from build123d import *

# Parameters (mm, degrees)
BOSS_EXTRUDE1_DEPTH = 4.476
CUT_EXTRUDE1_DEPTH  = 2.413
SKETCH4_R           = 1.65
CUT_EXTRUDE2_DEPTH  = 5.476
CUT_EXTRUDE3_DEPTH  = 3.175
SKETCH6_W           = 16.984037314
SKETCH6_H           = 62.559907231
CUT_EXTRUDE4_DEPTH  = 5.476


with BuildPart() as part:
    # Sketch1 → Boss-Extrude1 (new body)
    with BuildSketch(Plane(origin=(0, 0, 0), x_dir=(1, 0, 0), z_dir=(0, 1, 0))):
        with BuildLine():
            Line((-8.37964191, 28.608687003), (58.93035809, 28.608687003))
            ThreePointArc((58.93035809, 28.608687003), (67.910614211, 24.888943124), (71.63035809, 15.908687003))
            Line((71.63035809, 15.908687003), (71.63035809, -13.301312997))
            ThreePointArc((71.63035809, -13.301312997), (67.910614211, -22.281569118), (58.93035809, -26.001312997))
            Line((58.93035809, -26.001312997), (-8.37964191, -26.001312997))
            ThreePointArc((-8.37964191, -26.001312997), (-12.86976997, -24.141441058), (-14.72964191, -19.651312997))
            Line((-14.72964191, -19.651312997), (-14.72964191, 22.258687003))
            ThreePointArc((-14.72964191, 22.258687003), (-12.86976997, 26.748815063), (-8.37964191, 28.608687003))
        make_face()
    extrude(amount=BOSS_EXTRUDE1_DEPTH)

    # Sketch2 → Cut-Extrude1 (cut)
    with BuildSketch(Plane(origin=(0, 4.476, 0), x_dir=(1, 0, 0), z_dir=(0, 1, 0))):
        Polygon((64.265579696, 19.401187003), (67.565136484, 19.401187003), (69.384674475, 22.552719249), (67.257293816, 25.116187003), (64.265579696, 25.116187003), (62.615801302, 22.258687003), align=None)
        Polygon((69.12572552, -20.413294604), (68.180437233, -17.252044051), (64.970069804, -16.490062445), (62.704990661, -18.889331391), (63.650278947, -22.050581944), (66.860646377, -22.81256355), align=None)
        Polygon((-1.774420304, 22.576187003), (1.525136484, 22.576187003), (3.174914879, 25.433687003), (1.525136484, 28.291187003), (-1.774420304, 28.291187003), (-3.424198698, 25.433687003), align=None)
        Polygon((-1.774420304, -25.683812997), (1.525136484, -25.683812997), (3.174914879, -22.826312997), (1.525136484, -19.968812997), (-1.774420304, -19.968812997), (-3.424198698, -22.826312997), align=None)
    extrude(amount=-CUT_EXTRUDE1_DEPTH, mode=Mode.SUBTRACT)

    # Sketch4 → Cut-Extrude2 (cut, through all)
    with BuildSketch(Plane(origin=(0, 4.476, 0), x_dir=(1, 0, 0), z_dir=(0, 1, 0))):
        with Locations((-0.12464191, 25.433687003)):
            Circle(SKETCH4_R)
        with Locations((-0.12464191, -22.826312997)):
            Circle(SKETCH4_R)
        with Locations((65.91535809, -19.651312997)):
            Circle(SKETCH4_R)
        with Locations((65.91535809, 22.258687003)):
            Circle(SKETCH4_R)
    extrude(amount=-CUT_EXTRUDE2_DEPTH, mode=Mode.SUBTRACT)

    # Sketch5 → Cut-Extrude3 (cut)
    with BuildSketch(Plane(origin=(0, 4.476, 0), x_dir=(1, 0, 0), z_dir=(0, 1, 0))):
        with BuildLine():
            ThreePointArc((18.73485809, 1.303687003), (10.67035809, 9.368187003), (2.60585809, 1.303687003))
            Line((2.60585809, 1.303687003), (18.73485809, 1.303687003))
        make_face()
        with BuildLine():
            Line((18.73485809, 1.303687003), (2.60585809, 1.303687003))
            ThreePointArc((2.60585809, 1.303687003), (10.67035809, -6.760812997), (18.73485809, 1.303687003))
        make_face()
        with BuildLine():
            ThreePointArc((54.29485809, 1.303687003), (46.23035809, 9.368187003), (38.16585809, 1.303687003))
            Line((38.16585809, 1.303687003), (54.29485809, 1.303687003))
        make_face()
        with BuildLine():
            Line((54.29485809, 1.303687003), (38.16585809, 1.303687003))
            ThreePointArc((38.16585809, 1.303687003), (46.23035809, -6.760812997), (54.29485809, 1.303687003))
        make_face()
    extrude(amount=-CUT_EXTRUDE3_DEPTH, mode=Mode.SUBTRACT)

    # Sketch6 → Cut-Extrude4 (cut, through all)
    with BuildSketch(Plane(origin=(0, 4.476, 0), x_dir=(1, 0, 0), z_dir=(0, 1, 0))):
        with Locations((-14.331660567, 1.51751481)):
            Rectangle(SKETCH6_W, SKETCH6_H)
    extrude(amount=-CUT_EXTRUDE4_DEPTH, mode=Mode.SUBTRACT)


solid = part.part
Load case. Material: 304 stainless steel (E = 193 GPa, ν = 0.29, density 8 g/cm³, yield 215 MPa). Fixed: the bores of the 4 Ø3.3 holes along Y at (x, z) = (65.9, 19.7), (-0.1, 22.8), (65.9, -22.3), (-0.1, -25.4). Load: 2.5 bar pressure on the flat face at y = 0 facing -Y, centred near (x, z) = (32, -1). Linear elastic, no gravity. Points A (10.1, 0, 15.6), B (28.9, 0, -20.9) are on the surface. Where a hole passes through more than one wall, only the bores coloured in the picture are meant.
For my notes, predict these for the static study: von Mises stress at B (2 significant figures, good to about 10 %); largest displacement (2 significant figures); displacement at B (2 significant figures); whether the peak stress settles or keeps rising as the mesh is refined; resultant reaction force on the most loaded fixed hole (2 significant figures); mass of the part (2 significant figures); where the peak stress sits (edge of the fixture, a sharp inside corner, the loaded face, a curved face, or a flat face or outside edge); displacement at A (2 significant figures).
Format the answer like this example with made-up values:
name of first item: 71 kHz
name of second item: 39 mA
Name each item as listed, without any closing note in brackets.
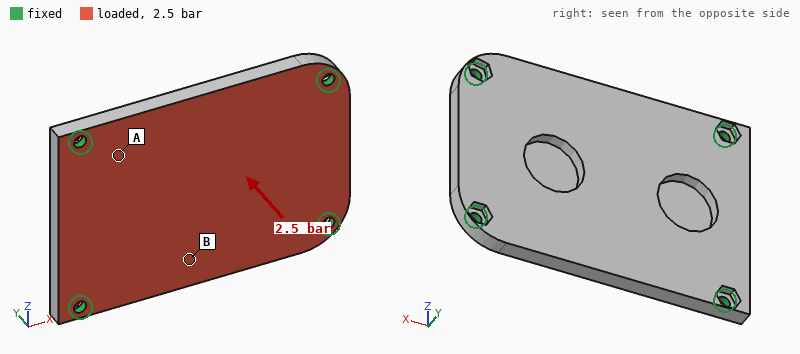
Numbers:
von Mises stress at B: 19 MPa
largest displacement: 24 µm
displacement at B: 21 µm
whether the peak stress settles or keeps rising as the mesh is refined: keeps rising
resultant reaction force on the most loaded fixed hole: 420 N
mass of the part: 140 g
where the peak stress sits: edge of the fixture
displacement at A: 11 µm
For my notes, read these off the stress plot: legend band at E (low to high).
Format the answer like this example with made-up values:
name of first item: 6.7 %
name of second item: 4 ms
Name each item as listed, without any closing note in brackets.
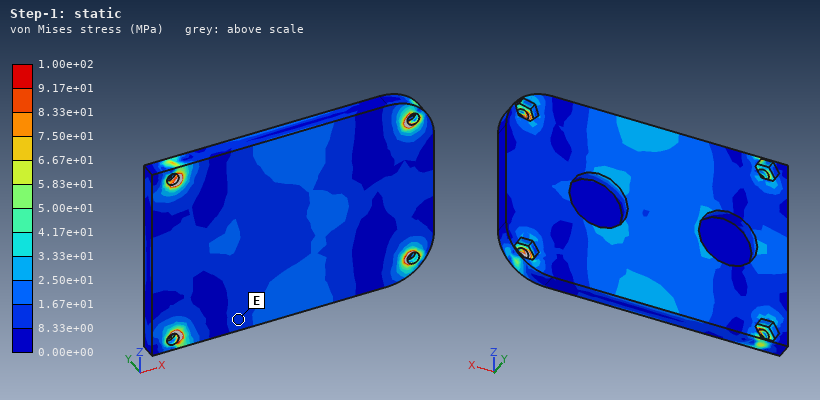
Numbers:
legend band at E: 8.33e+00 to 1.67e+01 MPa
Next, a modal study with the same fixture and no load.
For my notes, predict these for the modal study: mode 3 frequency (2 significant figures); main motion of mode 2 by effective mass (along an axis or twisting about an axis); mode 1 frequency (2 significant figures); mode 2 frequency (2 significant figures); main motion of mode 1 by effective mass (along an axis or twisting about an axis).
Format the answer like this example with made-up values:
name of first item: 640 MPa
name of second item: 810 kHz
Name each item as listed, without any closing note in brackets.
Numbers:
mode 3 frequency: 7400 Hz
main motion of mode 2 by effective mass: twisting about X
mode 1 frequency: 3300 Hz
mode 2 frequency: 5300 Hz
main motion of mode 1 by effective mass: along Y
